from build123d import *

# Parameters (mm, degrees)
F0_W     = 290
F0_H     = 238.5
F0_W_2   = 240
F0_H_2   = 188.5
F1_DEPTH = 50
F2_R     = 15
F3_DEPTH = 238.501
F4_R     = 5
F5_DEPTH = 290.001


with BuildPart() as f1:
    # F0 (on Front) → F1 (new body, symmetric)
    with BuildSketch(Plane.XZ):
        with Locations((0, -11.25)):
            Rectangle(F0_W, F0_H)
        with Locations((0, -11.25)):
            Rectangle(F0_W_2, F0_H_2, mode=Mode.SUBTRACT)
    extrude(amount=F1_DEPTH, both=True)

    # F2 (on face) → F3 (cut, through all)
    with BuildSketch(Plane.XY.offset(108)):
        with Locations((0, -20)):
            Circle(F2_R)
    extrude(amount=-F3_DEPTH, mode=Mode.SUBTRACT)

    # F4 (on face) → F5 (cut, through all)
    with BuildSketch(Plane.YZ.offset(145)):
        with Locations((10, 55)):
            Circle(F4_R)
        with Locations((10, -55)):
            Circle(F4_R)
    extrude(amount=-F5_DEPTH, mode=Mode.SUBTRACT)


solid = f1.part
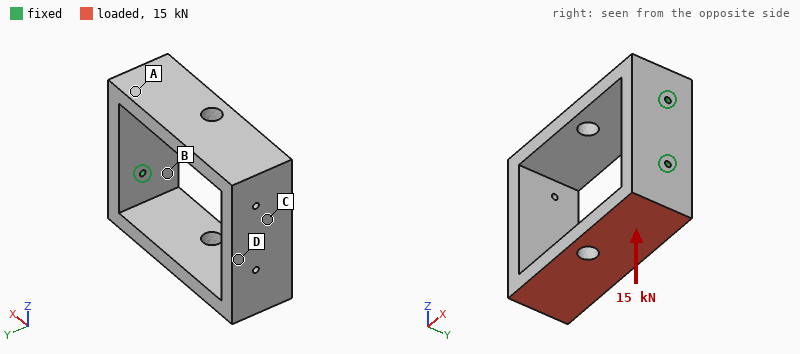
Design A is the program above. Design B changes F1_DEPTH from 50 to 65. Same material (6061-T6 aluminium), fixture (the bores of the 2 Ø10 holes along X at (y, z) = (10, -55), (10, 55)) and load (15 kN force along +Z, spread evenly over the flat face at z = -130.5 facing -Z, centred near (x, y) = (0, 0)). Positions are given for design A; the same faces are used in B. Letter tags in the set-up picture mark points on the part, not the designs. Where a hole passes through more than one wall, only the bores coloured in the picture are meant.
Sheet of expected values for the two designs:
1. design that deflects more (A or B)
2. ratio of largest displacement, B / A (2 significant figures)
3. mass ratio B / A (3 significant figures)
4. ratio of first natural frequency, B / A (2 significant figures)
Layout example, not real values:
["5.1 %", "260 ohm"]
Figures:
["A", "0.79", "1.31", "0.99"]
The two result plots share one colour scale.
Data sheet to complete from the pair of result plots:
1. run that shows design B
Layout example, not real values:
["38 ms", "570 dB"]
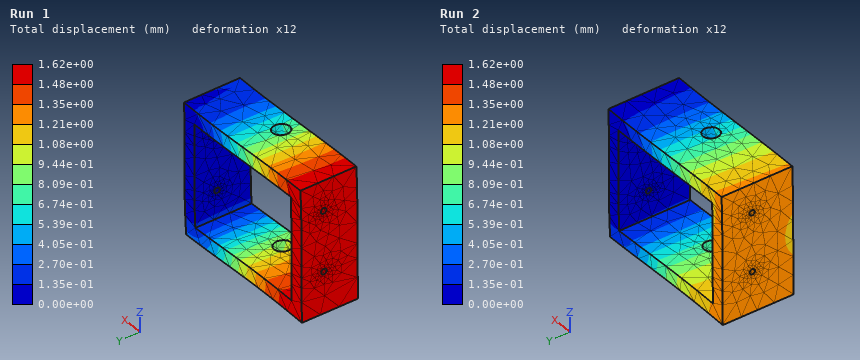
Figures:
["Run 2"]
